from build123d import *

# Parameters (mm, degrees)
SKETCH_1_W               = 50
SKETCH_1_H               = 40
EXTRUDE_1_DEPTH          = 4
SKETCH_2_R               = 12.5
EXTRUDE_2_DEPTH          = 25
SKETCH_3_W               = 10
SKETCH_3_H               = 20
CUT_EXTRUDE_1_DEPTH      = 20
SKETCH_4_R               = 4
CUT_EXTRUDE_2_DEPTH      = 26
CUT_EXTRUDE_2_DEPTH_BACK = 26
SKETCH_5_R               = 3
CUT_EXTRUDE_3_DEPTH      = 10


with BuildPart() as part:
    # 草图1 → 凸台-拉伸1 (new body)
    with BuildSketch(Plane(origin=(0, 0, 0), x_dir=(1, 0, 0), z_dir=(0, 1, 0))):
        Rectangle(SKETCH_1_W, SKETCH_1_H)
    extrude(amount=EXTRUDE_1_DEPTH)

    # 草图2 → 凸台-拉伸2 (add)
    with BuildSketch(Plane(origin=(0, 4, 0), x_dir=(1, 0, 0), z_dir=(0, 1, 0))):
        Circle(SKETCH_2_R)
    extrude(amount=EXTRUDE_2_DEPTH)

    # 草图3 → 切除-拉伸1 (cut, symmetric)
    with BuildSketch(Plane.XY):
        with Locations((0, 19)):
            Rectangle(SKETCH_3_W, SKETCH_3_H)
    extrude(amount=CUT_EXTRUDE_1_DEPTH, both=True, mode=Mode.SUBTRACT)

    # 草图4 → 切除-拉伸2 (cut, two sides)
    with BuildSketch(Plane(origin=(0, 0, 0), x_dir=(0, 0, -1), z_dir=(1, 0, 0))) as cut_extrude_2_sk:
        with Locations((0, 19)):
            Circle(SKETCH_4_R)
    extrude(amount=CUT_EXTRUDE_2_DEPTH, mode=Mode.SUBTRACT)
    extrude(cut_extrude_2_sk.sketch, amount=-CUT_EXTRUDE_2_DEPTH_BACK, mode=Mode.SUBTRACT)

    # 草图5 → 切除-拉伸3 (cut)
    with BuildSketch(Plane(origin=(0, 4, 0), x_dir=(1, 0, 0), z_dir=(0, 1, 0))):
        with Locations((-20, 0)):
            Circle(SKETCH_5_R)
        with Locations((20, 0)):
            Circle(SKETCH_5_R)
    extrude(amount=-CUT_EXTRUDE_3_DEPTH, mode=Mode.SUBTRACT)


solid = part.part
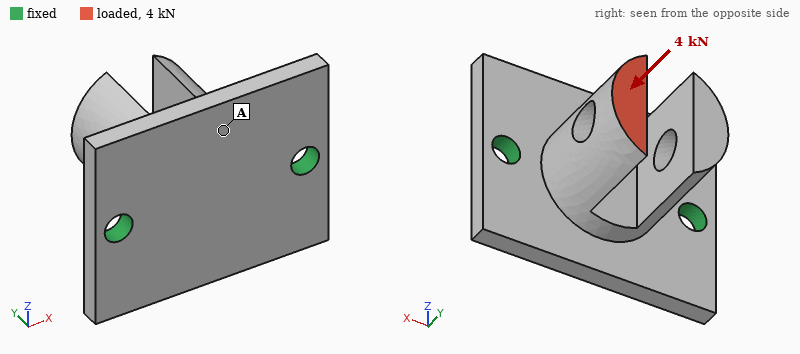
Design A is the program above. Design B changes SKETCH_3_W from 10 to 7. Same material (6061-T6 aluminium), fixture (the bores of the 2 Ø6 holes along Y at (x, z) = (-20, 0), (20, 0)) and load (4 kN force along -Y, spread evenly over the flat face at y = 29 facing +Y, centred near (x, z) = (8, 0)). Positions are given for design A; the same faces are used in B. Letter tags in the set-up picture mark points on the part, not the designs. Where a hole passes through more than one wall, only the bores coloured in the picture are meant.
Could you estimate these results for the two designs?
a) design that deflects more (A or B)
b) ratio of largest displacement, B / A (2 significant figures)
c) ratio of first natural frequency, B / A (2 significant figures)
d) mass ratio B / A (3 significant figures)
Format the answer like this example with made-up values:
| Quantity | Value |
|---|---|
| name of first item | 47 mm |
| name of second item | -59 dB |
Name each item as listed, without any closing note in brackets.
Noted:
| Quantity | Value |
|---|---|
| design that deflects more | A |
| ratio of largest displacement, B / A | 0.86 |
| ratio of first natural frequency, B / A | 0.91 |
| mass ratio B / A | 1.09 |
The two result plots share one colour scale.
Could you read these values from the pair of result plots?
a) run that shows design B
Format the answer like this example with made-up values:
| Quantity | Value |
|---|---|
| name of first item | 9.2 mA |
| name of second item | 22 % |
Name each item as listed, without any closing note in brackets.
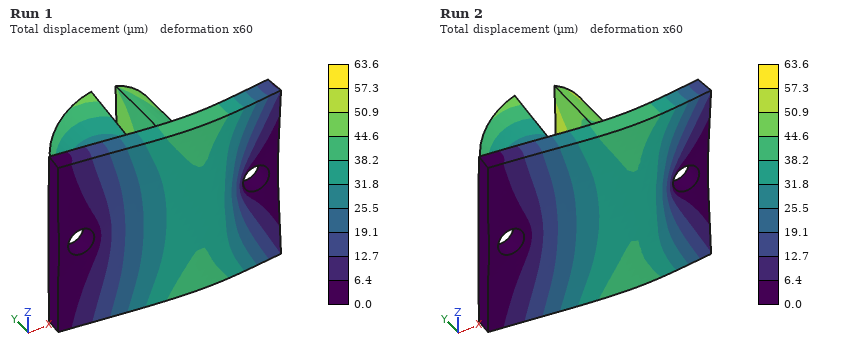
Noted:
| Quantity | Value |
|---|---|
| run that shows design B | Run 1 |
